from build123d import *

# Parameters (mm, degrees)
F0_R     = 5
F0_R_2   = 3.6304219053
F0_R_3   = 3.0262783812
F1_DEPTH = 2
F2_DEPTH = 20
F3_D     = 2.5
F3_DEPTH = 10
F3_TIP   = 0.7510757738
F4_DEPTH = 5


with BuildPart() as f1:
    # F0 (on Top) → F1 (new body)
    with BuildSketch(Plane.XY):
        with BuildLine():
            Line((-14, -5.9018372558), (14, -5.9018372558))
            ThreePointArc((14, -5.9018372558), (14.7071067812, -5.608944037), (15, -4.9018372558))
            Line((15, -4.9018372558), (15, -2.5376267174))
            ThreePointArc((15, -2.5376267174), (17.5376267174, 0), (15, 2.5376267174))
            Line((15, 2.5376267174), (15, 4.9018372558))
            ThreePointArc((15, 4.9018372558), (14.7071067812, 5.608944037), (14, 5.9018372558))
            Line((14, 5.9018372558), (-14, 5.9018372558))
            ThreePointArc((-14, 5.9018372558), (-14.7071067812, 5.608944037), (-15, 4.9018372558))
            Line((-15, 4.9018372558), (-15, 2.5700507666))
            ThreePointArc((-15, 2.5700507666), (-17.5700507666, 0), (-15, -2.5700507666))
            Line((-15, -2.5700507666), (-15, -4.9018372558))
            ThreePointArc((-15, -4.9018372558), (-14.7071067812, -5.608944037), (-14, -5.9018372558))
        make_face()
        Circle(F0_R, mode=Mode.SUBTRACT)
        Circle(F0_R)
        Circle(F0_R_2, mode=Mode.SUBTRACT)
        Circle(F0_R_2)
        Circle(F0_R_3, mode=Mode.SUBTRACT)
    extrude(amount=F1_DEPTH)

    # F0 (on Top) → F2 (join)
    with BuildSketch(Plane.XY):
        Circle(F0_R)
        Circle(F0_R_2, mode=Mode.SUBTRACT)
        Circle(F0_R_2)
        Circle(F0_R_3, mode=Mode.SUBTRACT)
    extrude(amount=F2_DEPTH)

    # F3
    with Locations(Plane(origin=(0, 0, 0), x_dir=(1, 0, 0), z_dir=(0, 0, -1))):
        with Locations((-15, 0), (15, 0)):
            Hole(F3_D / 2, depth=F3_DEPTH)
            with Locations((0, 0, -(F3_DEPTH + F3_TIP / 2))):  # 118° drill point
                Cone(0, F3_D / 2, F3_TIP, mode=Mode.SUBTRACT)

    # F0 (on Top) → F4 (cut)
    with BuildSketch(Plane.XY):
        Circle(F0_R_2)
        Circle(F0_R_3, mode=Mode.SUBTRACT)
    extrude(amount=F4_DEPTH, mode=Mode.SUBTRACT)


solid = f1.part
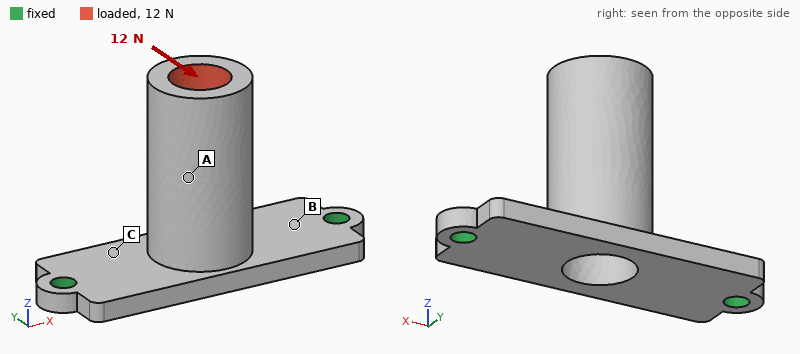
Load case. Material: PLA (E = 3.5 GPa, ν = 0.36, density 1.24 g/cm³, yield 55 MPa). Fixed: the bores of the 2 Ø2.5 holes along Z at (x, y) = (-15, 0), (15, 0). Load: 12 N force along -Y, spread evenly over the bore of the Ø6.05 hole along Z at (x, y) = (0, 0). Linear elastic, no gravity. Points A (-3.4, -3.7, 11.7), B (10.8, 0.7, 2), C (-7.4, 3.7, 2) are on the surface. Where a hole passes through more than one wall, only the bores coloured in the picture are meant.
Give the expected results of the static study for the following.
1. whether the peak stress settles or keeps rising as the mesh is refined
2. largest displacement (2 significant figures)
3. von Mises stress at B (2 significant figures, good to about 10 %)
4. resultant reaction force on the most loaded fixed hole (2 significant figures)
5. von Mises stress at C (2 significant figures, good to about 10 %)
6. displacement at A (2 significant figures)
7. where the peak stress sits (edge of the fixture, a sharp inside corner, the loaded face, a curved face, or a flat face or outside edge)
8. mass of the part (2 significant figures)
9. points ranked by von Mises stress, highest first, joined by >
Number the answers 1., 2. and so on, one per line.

1. keeps rising
2. 0.43 mm
3. 9.0 MPa
4. 6.0 N
5. 6.7 MPa
6. 0.25 mm
7. edge of the fixture
8. 1.9 g
9. B > C > A
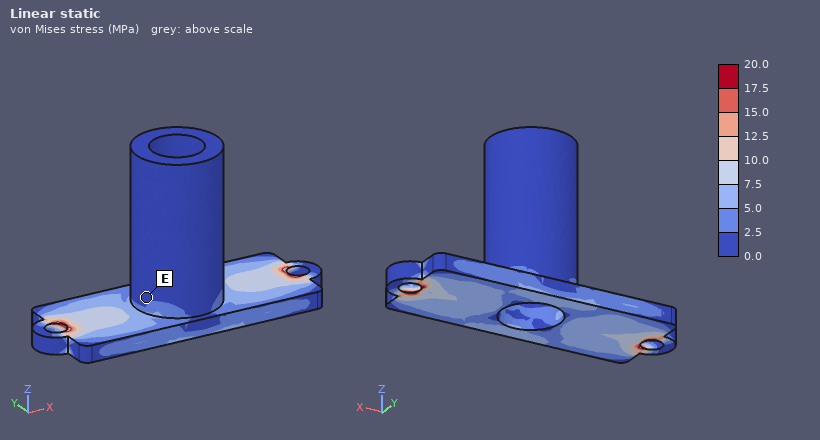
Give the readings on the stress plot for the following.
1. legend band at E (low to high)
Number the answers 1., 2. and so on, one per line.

1. 0.0 to 2.5 MPa
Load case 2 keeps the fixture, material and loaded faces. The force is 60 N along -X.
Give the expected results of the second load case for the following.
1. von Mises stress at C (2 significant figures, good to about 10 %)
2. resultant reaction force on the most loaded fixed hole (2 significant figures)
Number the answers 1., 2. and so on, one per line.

1. 13 MPa
2. 44 N
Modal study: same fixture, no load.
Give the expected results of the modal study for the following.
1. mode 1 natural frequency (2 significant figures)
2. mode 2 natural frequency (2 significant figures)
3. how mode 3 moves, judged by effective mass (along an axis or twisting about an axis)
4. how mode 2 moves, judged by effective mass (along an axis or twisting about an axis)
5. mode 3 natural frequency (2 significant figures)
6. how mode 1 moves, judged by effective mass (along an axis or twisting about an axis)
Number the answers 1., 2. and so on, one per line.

1. 1000 Hz
2. 2200 Hz
3. along Z
4. along X
5. 2400 Hz
6. along Y
